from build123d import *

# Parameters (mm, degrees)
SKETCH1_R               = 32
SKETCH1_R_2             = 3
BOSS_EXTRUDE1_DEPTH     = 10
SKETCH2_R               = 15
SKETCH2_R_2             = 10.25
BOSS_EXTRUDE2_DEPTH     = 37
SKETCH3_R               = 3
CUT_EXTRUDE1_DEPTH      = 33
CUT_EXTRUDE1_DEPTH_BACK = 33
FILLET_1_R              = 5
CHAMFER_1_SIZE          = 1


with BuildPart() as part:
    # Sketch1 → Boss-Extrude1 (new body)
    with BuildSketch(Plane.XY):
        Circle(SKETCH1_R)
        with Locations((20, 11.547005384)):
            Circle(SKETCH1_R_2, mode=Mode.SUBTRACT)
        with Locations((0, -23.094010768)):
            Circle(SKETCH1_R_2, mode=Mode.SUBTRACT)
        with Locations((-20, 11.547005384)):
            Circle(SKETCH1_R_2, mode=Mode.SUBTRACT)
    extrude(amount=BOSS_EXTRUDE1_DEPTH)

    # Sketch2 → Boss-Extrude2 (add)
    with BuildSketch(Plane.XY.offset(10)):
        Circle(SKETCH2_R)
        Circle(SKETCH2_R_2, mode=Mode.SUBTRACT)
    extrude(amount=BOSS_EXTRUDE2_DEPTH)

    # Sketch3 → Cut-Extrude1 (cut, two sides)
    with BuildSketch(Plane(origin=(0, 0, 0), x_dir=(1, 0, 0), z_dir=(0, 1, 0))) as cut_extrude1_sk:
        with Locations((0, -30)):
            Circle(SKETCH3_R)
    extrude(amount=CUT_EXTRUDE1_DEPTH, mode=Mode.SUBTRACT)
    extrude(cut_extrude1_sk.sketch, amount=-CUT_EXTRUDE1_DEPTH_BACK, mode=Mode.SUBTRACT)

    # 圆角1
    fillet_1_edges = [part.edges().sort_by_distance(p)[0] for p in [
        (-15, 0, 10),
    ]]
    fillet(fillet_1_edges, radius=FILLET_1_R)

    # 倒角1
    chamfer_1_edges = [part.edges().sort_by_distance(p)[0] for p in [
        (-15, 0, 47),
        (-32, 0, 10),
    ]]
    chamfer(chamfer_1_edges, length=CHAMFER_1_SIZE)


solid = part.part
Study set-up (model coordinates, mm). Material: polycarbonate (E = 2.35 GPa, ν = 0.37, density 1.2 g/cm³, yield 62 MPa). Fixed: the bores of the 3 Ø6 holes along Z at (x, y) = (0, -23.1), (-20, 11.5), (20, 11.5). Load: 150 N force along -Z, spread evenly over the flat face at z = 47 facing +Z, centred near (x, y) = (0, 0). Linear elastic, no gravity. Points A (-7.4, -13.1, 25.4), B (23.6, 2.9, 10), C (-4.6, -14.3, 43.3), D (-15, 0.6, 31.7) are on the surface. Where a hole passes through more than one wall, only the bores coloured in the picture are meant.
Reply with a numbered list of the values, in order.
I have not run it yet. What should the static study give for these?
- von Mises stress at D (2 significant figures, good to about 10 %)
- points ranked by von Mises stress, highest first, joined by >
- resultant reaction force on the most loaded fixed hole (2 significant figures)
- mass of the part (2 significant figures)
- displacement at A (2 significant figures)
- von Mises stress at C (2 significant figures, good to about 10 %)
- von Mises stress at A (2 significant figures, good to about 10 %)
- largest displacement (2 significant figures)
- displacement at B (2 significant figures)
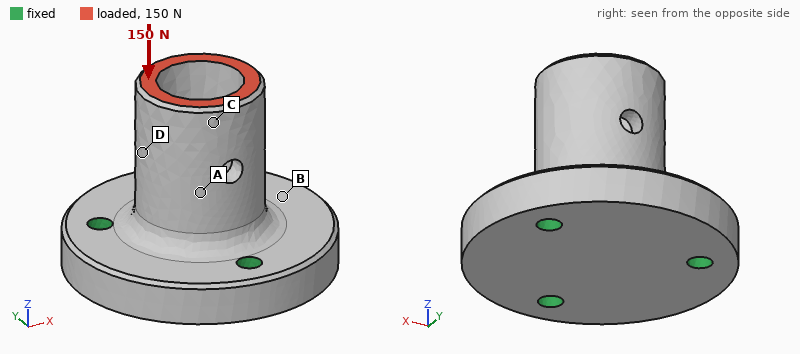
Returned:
1. 0.35 MPa
2. A > D > C > B
3. 52 N
4. 54 g
5. 6.4 µm
6. 0.24 MPa
7. 0.47 MPa
8. 11 µm
9. 1.7 µm
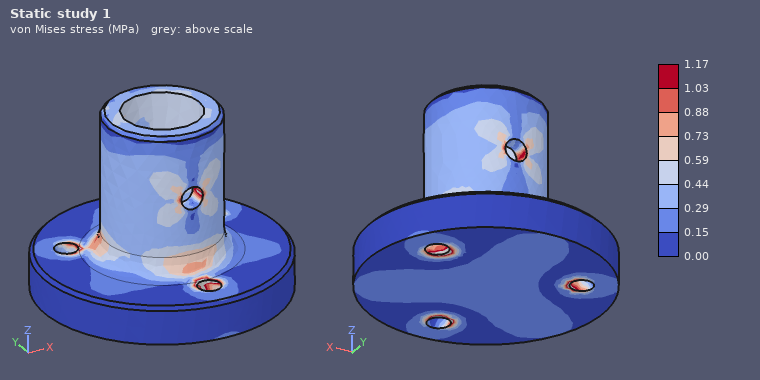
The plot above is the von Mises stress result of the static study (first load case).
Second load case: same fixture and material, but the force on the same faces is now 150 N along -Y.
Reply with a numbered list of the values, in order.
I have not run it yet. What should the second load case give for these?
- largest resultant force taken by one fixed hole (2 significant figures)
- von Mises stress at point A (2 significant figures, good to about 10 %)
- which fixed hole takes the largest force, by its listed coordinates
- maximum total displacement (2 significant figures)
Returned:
1. 180 N
2. 1.7 MPa
3. (0, -23.1)
4. 0.11 mm
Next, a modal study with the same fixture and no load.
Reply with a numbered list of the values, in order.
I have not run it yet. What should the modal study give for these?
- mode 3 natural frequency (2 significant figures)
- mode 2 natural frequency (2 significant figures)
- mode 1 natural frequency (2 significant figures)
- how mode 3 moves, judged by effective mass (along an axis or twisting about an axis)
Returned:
1. 4500 Hz
2. 2600 Hz
3. 2600 Hz
4. along Z
